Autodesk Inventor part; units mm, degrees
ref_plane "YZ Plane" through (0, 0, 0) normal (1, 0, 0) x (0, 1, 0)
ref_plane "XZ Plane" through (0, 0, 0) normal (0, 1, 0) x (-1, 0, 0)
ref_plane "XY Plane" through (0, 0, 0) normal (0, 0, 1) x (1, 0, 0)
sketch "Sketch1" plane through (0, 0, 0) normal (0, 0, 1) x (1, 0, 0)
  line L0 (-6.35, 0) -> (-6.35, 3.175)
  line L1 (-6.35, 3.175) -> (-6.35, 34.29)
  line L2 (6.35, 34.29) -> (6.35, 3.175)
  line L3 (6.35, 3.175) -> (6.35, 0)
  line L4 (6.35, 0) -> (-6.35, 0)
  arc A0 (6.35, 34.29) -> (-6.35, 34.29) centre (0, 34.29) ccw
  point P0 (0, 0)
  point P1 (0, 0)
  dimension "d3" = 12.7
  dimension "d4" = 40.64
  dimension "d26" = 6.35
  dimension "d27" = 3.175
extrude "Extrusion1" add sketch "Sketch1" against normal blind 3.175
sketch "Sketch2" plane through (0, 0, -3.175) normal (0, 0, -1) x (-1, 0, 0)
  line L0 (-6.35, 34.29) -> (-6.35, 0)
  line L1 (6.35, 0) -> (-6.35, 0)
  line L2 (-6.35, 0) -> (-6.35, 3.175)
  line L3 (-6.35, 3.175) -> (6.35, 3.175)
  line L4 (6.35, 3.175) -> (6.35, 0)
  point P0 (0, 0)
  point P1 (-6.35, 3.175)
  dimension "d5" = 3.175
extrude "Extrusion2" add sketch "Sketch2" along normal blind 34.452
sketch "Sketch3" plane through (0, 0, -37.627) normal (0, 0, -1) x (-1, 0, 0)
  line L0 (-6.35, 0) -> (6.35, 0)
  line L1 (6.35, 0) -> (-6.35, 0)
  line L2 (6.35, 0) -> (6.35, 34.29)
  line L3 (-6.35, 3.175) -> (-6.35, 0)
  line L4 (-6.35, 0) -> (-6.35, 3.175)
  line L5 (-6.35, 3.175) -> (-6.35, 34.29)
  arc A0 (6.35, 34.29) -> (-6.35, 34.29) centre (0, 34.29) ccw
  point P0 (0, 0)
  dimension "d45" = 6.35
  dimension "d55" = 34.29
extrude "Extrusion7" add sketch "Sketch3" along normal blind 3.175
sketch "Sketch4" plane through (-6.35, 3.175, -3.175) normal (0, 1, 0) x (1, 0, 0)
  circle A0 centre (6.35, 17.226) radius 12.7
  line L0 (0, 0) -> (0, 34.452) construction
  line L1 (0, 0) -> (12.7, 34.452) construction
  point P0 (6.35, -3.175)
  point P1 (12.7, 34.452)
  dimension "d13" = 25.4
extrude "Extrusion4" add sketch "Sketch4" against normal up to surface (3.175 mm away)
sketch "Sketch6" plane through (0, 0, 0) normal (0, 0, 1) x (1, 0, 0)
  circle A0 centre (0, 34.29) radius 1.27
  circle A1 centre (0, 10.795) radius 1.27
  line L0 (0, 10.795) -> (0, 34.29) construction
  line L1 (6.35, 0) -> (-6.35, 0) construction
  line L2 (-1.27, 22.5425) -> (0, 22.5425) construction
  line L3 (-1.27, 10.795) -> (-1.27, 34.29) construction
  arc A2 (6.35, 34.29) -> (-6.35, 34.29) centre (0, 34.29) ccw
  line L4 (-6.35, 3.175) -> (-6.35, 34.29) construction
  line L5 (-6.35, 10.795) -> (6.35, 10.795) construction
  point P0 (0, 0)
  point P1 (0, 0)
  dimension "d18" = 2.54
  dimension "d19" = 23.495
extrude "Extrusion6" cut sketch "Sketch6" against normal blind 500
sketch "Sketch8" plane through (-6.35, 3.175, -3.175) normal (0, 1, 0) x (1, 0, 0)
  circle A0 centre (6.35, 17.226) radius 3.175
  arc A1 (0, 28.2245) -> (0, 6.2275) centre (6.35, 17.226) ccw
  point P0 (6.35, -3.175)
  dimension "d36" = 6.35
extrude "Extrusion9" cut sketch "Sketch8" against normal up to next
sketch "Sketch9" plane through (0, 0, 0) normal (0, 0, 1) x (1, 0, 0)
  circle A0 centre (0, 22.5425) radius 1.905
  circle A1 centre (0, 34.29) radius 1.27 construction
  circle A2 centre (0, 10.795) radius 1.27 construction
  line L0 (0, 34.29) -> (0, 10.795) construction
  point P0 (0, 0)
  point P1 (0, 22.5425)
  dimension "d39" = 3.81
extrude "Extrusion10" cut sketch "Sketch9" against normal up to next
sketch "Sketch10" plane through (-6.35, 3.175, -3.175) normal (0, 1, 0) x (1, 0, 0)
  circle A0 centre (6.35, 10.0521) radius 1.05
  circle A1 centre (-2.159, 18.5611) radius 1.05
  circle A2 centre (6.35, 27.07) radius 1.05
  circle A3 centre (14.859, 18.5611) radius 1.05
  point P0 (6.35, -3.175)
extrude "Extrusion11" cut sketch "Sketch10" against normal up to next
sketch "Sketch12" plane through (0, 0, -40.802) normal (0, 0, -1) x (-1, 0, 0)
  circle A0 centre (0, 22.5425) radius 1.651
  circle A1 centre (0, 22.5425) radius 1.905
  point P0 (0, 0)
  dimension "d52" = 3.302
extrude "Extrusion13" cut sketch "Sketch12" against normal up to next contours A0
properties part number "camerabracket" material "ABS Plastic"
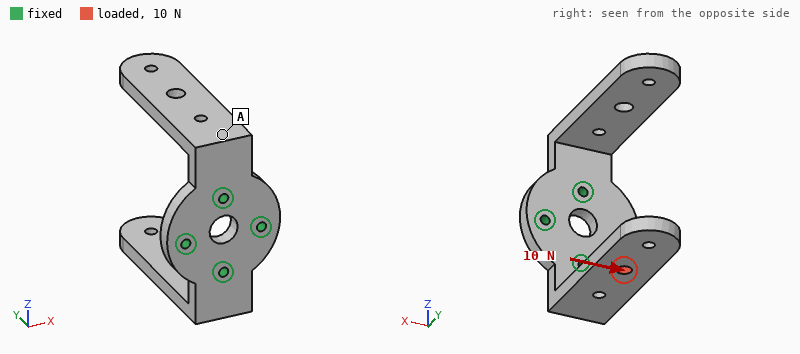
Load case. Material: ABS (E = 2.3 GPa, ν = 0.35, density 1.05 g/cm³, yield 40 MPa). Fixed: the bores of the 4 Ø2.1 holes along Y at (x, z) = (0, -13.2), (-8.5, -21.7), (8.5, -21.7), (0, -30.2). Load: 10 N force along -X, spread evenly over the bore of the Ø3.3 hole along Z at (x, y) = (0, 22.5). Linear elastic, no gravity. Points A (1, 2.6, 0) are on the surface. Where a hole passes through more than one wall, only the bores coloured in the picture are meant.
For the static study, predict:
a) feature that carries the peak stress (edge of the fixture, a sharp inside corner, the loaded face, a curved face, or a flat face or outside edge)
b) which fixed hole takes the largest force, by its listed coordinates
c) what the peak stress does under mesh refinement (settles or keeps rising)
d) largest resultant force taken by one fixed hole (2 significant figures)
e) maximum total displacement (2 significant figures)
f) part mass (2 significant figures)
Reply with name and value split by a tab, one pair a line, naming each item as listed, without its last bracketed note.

feature that carries the peak stress	edge of the fixture
which fixed hole takes the largest force, by its listed coordinates	(0, -30.2)
what the peak stress does under mesh refinement	keeps rising
largest resultant force taken by one fixed hole	9.2 N
maximum total displacement	0.64 mm
part mass	5.2 g
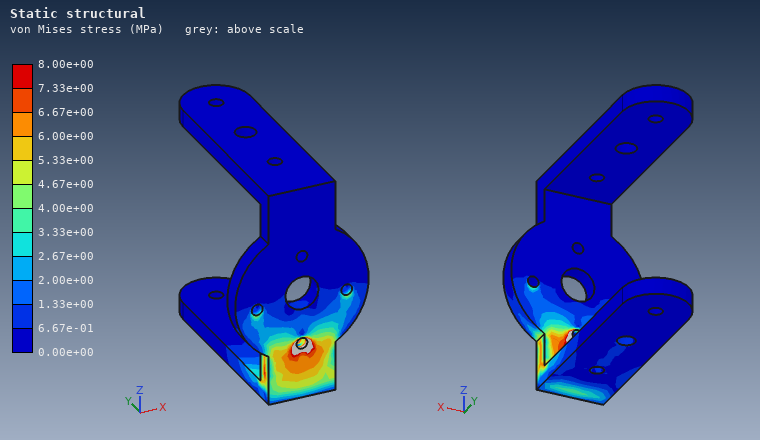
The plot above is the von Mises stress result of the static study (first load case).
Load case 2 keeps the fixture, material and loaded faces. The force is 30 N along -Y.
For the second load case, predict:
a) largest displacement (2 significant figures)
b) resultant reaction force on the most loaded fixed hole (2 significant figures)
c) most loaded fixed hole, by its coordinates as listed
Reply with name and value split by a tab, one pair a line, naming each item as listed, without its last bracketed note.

largest displacement	0.63 mm
resultant reaction force on the most loaded fixed hole	41 N
most loaded fixed hole, by its coordinates as listed	(0, -30.2)
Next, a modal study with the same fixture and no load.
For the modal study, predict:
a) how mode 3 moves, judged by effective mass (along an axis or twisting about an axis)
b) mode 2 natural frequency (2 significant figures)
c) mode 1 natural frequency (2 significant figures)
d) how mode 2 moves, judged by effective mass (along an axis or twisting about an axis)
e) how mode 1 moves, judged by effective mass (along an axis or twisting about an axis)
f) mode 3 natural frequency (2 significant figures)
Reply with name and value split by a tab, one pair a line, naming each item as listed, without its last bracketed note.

how mode 3 moves, judged by effective mass	along X
mode 2 natural frequency	400 Hz
mode 1 natural frequency	370 Hz
how mode 2 moves, judged by effective mass	along Z
how mode 1 moves, judged by effective mass	along Z
mode 3 natural frequency	590 Hz
